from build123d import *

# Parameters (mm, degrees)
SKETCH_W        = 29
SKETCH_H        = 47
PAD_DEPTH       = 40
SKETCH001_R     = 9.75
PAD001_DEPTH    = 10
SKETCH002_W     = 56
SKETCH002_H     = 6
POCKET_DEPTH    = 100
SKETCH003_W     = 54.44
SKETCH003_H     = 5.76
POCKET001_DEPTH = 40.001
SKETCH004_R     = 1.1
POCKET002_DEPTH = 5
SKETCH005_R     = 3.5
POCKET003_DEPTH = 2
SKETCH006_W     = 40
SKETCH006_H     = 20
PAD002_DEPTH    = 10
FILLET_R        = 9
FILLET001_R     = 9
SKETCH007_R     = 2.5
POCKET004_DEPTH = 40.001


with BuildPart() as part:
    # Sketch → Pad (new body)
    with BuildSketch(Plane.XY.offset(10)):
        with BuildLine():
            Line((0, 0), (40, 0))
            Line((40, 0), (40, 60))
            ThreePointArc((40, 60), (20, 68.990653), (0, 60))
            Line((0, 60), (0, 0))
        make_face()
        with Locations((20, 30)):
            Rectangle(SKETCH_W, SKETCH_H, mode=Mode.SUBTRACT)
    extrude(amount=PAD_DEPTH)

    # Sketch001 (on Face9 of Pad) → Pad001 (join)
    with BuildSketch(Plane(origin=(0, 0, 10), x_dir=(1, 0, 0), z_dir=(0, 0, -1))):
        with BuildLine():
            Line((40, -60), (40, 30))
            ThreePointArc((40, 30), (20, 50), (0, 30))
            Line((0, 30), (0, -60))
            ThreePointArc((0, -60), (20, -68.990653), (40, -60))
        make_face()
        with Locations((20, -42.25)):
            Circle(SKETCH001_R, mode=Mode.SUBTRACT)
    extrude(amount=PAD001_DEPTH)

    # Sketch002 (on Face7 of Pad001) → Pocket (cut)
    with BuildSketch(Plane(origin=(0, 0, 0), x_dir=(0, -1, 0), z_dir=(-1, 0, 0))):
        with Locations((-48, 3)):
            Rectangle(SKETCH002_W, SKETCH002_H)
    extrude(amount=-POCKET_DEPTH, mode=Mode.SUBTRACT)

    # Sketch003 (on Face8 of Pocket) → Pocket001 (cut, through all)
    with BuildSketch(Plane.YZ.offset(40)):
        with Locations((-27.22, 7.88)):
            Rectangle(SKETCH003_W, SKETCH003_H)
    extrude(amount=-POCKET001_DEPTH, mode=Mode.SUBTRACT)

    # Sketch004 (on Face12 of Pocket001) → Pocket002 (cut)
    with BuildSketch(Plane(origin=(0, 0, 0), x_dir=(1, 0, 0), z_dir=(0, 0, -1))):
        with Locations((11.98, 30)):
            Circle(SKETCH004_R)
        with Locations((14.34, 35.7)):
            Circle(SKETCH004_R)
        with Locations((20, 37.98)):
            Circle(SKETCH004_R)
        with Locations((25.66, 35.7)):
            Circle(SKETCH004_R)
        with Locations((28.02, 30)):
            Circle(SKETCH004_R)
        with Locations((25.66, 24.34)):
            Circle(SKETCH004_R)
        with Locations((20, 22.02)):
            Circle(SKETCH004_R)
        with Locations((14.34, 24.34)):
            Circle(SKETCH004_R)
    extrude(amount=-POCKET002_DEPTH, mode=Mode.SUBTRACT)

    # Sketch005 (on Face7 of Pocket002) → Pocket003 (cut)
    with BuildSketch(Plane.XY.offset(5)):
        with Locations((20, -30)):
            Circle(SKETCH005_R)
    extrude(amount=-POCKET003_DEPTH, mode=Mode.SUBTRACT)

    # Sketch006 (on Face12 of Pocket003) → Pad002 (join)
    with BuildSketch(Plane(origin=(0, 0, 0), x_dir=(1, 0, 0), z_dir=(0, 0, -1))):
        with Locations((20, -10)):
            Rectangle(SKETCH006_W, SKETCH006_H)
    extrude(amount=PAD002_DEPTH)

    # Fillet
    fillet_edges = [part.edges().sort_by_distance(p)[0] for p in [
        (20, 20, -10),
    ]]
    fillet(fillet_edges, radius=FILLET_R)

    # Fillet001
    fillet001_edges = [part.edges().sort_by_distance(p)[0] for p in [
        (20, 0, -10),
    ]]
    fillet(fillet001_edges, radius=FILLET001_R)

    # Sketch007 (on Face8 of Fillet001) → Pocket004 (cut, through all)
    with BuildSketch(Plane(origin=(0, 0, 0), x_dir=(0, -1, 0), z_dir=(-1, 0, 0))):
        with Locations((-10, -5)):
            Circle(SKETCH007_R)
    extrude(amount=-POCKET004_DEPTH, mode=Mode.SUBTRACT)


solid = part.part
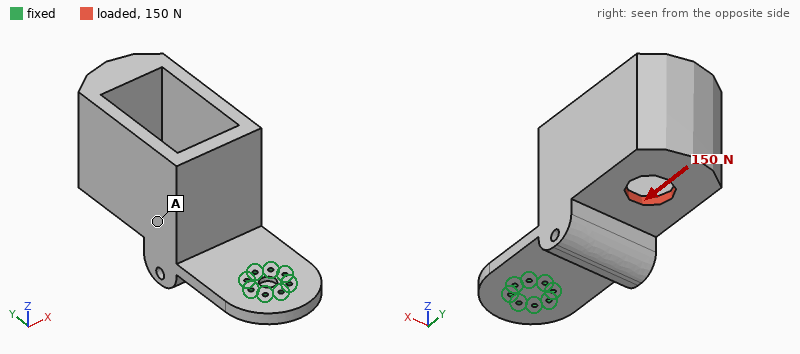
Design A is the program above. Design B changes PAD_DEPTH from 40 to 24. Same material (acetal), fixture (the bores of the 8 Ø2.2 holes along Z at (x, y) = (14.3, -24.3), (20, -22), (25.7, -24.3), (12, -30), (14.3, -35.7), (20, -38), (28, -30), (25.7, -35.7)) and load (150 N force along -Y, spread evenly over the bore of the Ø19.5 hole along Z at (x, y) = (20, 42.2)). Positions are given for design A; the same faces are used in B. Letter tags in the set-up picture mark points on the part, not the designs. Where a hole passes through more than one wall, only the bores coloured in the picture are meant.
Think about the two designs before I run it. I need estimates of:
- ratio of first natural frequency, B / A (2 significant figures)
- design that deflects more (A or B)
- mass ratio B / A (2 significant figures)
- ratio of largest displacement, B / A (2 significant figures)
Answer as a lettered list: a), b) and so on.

a) 1.3
b) A
c) 0.74
d) 0.92
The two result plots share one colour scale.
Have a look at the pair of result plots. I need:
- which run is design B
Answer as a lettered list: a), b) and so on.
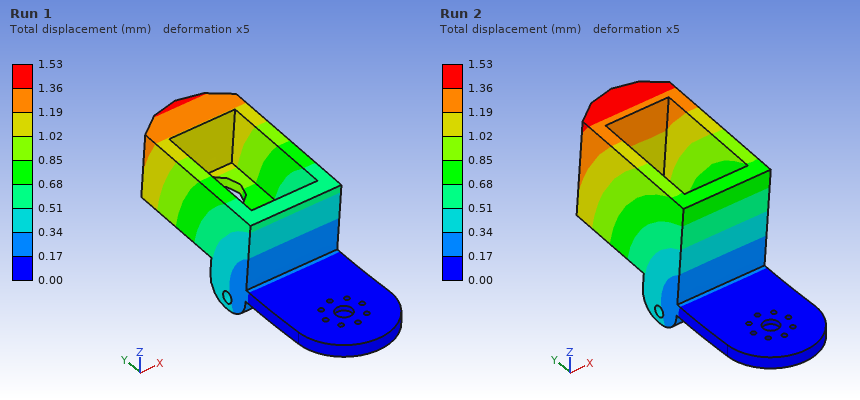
a) Run 1
